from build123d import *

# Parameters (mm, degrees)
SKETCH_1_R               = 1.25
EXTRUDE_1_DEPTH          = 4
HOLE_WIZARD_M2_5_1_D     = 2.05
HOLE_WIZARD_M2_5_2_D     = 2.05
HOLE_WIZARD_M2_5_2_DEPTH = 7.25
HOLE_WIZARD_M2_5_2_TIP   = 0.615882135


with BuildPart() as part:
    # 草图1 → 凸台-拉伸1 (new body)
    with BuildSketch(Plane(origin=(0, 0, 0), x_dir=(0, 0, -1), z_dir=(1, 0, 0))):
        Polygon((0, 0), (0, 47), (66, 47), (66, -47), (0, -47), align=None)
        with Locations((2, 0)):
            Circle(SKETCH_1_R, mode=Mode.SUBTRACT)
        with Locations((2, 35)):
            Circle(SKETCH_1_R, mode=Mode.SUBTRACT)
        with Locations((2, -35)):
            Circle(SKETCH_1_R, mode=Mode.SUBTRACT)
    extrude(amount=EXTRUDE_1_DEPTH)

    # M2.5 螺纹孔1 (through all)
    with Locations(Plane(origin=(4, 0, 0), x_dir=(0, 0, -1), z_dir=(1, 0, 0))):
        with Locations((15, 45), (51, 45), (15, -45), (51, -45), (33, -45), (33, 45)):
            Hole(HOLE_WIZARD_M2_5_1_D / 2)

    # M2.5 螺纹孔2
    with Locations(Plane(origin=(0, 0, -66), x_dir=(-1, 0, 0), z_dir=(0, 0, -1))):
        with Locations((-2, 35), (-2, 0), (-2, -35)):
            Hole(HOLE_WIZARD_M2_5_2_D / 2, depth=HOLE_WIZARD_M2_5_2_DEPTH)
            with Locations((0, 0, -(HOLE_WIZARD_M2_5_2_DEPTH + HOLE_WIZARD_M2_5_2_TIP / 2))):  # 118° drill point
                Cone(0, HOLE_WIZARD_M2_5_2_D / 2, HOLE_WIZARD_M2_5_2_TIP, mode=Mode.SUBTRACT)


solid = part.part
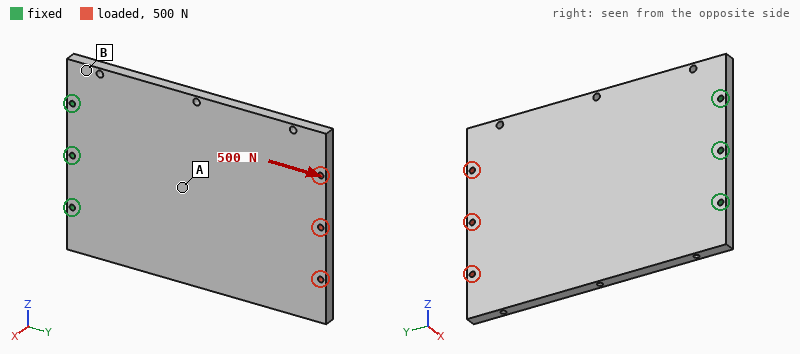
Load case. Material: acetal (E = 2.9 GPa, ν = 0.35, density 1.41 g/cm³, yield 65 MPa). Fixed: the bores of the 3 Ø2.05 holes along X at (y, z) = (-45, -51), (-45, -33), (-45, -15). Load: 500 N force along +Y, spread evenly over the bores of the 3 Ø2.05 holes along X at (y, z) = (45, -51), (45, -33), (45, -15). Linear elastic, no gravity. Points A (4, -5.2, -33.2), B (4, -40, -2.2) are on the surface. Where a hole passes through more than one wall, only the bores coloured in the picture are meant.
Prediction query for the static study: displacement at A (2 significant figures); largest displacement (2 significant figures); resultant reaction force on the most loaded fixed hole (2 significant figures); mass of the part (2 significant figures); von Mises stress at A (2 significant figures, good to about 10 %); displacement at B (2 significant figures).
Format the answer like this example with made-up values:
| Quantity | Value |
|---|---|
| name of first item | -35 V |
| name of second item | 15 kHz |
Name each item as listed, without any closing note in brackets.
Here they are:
| Quantity | Value |
|---|---|
| displacement at A | 37 µm |
| largest displacement | 93 µm |
| resultant reaction force on the most loaded fixed hole | 170 N |
| mass of the part | 35 g |
| von Mises stress at A | 2.2 MPa |
| displacement at B | 25 µm |
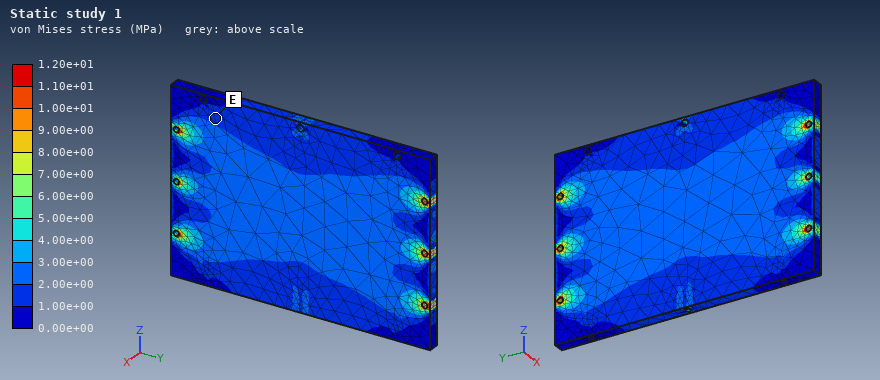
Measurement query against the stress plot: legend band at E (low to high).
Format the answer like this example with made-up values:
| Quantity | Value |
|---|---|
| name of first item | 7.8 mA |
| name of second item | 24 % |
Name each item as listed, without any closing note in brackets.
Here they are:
| Quantity | Value |
|---|---|
| legend band at E | 1.00e+00 to 2.00e+00 MPa |
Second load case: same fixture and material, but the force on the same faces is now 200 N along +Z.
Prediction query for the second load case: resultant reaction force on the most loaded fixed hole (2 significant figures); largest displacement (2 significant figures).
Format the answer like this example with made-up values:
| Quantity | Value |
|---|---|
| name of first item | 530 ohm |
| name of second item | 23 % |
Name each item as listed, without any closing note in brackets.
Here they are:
| Quantity | Value |
|---|---|
| resultant reaction force on the most loaded fixed hole | 490 N |
| largest displacement | 0.54 mm |
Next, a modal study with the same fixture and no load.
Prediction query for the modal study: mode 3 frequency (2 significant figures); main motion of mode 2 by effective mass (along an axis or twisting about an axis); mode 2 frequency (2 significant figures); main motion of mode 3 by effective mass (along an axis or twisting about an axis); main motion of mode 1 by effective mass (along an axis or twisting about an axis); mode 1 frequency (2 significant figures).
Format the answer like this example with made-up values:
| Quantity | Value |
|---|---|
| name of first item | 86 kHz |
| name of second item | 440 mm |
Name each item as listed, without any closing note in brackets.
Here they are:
| Quantity | Value |
|---|---|
| mode 3 frequency | 630 Hz |
| main motion of mode 2 by effective mass | twisting about Y |
| mode 2 frequency | 320 Hz |
| main motion of mode 3 by effective mass | along X |
| main motion of mode 1 by effective mass | along X |
| mode 1 frequency | 100 Hz |
